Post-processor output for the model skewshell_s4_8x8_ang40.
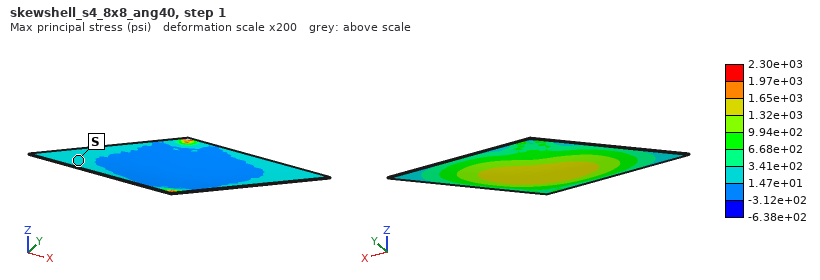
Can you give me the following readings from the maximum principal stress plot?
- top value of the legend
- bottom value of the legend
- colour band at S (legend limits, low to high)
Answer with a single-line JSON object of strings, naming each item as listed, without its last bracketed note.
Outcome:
{"top value of the legend": "2.30e+03 psi", "bottom value of the legend": "-6.38e+02 psi", "colour band at S": "1.47e+01 to 3.41e+02 psi"}
